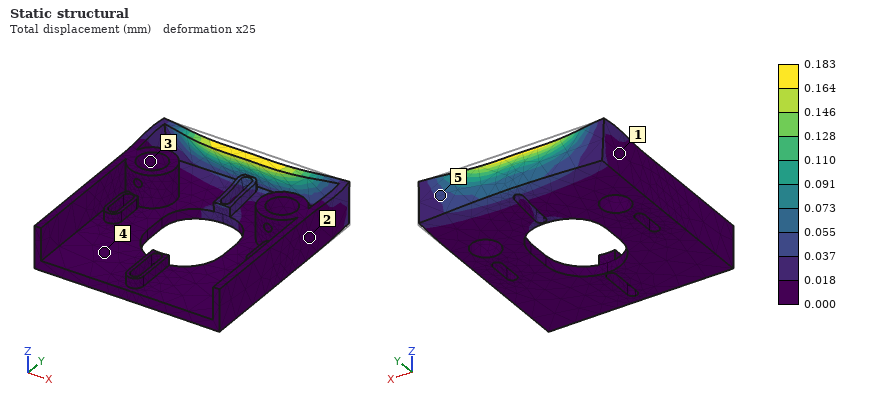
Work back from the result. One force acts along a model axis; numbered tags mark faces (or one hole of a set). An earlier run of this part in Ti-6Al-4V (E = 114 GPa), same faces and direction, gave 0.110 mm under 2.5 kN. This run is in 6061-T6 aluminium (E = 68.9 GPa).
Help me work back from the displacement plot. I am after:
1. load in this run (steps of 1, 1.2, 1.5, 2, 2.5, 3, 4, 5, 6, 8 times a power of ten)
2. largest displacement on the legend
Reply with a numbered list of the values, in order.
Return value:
1. 2.5 kN
2. 0.183 mm
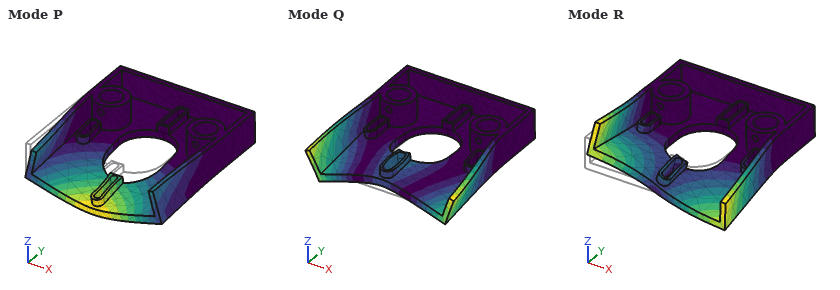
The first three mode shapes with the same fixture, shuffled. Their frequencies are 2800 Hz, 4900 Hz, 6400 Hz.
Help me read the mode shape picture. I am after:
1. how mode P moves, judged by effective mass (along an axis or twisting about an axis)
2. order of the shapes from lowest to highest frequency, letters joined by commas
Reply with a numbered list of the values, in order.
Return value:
1. along Z
2. P, R, Q
